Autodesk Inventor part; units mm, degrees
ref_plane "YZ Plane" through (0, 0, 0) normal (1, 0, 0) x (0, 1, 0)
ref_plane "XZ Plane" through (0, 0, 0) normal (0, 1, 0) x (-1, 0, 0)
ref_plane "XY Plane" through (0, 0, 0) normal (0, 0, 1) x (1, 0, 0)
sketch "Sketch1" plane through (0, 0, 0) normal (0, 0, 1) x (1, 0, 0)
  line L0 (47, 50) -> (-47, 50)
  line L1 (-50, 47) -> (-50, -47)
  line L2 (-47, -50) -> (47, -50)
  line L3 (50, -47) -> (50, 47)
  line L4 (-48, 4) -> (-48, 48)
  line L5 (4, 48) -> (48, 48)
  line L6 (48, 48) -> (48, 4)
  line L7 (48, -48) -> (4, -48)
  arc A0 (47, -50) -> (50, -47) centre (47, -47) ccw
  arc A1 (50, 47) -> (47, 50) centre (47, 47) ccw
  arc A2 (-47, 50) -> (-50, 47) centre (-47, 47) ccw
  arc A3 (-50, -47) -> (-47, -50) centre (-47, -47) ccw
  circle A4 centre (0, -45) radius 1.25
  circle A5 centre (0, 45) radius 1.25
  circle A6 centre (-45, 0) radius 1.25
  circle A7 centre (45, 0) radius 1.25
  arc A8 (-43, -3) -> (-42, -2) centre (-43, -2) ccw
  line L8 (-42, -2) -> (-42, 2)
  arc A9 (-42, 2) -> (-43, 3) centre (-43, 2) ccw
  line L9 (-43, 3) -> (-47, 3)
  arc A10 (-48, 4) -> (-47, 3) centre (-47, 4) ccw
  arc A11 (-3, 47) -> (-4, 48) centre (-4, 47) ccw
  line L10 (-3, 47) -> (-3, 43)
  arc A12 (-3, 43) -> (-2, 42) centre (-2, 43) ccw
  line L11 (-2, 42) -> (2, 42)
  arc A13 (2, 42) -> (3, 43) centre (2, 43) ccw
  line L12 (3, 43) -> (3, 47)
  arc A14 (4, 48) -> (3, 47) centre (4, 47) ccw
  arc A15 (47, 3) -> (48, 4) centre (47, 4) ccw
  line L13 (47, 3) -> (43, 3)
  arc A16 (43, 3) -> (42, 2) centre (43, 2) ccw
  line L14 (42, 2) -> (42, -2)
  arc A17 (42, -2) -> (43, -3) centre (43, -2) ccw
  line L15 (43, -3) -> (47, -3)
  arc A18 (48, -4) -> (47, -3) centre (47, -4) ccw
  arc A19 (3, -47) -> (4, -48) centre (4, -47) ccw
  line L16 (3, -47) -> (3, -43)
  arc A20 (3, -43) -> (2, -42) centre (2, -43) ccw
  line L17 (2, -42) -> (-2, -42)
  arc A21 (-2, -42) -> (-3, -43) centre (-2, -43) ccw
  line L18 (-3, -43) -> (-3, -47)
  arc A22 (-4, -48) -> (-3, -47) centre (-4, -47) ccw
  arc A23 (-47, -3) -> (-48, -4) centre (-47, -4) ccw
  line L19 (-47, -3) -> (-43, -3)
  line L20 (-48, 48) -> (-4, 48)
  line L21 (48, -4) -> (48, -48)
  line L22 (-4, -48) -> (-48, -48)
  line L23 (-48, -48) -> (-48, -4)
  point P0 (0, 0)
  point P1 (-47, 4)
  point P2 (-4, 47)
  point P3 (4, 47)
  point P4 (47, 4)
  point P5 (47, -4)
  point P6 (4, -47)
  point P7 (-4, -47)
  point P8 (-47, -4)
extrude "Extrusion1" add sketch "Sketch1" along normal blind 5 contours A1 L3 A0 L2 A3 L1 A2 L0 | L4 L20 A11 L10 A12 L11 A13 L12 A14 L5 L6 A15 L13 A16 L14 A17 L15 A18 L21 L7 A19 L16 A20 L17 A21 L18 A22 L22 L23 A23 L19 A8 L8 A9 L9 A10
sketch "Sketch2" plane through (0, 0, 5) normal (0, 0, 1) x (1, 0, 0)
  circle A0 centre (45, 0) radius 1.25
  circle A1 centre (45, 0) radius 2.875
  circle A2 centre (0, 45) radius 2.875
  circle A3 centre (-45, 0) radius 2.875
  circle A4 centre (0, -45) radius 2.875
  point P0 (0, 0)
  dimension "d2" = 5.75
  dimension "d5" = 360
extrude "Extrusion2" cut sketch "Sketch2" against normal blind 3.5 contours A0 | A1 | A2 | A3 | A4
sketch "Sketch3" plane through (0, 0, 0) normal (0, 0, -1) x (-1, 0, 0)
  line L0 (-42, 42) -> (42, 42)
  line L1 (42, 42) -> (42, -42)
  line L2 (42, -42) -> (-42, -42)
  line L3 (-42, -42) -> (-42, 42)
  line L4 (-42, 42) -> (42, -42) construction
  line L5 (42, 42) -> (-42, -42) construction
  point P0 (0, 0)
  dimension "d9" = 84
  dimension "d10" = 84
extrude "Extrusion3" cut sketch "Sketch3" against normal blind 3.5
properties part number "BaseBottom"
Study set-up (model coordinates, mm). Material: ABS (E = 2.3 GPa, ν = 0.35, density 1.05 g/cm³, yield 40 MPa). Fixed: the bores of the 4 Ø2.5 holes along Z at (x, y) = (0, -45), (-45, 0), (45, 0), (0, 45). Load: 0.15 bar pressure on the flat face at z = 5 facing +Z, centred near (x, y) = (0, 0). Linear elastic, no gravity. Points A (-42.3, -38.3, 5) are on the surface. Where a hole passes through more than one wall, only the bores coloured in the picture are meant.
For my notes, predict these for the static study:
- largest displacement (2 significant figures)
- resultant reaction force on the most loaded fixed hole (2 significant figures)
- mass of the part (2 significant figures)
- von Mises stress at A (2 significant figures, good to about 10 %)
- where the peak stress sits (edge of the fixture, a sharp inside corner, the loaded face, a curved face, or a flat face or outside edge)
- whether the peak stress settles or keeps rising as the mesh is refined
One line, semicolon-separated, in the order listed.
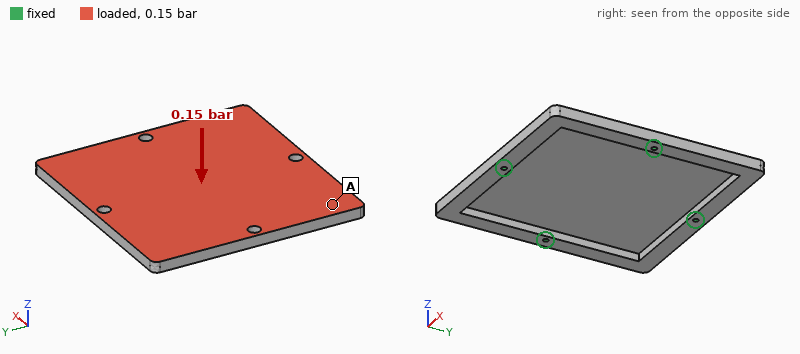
1.5 mm; 57 N; 26 g; 1.6 MPa; edge of the fixture; keeps rising
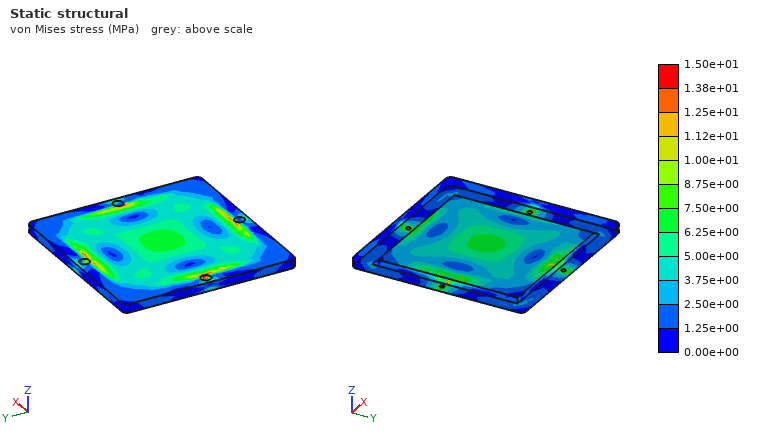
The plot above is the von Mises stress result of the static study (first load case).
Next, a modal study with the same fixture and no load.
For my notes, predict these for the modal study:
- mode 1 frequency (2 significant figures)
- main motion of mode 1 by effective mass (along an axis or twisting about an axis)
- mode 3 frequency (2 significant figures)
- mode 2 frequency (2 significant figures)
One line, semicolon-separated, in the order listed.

500 Hz; along Z; 550 Hz; 550 Hz
